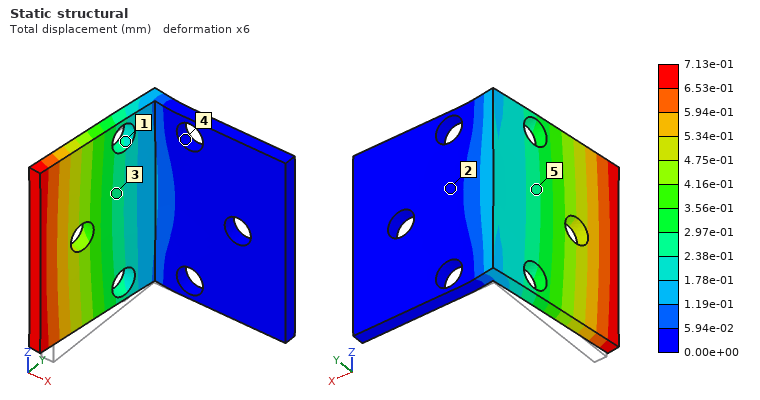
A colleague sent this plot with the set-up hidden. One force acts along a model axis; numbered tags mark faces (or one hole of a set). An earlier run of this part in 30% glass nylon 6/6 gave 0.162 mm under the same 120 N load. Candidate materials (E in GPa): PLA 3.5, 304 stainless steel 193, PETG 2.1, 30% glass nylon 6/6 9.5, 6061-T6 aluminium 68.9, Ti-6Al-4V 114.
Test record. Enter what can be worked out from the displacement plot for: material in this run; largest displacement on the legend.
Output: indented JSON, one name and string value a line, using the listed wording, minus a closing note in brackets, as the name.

{
  "material in this run": "PETG",
  "largest displacement on the legend": "7.13e-01 mm"
}
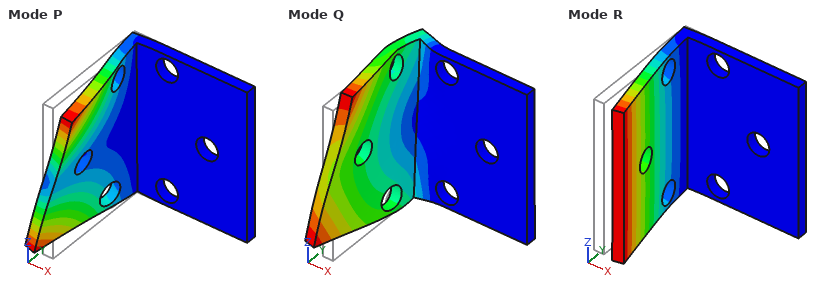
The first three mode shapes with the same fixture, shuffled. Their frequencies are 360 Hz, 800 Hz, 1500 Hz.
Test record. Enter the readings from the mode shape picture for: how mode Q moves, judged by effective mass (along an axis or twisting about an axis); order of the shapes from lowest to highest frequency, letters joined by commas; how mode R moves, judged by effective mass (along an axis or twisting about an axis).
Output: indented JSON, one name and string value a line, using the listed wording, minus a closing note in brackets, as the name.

{
  "how mode Q moves, judged by effective mass": "along Z",
  "order of the shapes from lowest to highest frequency, letters joined by commas": "R, P, Q",
  "how mode R moves, judged by effective mass": "along X"
}
